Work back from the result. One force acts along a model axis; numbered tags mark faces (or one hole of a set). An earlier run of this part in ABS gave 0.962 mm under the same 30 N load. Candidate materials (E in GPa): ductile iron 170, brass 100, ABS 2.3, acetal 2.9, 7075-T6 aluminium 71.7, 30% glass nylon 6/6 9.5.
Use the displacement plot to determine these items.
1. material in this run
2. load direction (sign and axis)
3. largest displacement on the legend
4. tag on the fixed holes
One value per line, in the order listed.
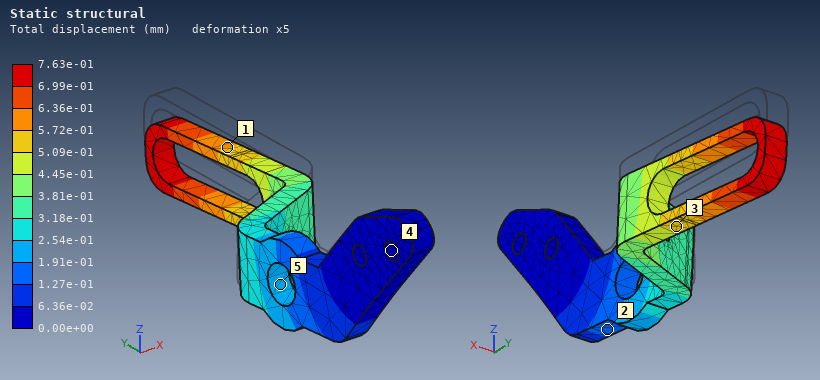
acetal
-Z
7.63e-01 mm
4
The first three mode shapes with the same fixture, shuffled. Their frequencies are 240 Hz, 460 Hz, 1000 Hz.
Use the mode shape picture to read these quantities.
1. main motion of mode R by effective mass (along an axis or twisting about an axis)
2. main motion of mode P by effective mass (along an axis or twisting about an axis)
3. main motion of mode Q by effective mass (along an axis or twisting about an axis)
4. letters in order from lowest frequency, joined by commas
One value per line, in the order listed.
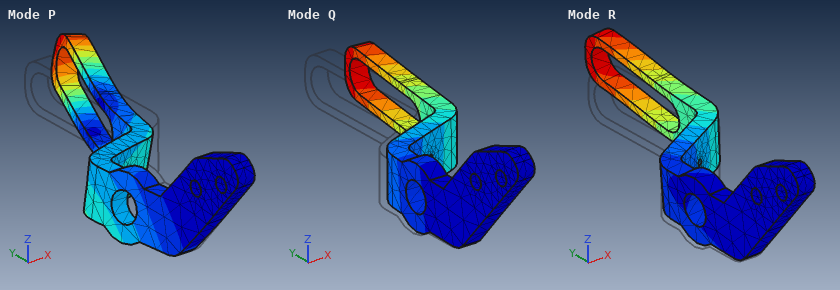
along Z
along X
along X
Q, R, P
